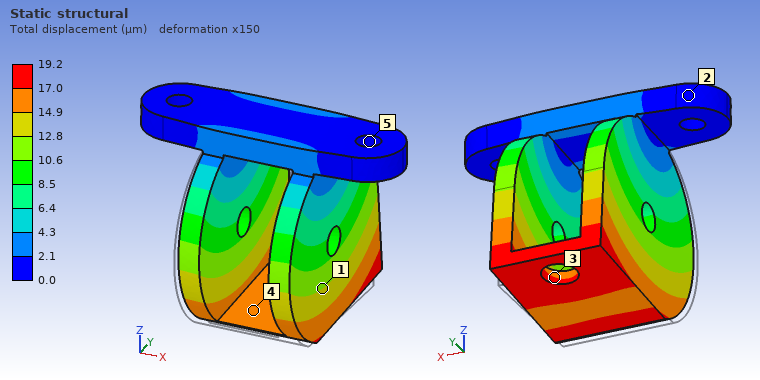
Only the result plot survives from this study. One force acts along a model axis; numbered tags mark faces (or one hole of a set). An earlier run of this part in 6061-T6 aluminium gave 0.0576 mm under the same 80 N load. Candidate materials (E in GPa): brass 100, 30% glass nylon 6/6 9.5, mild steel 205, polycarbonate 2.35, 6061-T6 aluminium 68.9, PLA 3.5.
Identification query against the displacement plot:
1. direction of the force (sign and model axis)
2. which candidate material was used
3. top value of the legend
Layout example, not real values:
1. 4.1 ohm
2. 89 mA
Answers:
1. +Y
2. mild steel
3. 19.2 µm
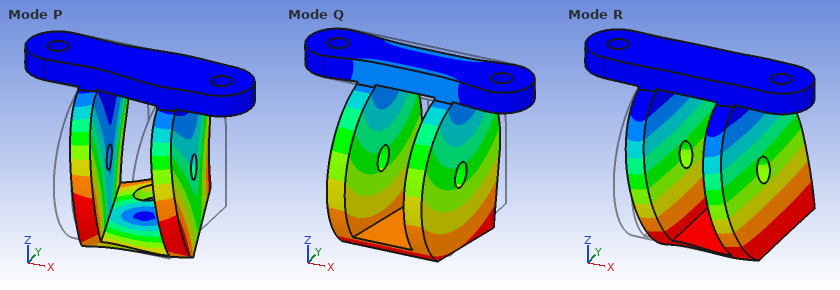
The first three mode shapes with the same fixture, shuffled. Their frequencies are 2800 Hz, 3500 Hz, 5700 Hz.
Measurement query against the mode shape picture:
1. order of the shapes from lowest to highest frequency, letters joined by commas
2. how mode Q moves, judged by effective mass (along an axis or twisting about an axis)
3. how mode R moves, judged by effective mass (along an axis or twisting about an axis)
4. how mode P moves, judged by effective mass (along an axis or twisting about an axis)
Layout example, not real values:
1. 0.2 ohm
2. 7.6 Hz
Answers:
1. Q, R, P
2. along Y
3. along X
4. twisting about Z
